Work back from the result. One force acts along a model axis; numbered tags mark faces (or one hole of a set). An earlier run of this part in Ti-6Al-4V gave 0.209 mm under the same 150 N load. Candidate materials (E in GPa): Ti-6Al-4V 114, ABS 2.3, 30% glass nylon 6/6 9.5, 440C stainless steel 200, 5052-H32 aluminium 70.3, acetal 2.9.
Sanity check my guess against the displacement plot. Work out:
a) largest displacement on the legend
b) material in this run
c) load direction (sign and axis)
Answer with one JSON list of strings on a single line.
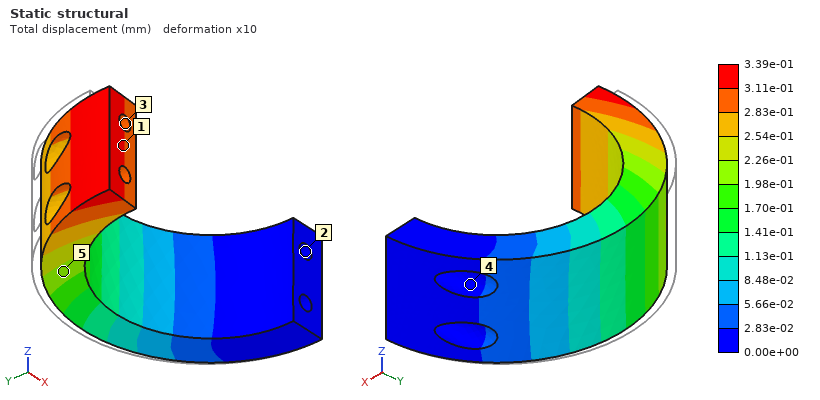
["3.39e-01 mm", "5052-H32 aluminium", "-Y"]
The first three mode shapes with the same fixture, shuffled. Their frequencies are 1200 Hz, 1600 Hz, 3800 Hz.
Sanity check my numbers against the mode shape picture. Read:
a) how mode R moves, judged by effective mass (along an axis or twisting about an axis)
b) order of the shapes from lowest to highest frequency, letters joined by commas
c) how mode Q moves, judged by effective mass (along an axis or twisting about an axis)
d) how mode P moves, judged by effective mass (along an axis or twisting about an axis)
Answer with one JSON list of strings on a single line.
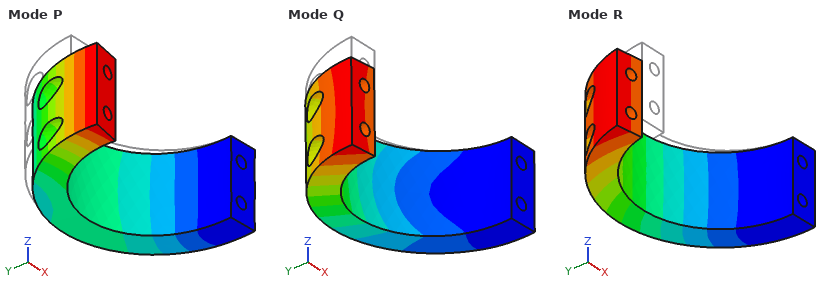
["along Y", "R, Q, P", "along Z", "along X"]
